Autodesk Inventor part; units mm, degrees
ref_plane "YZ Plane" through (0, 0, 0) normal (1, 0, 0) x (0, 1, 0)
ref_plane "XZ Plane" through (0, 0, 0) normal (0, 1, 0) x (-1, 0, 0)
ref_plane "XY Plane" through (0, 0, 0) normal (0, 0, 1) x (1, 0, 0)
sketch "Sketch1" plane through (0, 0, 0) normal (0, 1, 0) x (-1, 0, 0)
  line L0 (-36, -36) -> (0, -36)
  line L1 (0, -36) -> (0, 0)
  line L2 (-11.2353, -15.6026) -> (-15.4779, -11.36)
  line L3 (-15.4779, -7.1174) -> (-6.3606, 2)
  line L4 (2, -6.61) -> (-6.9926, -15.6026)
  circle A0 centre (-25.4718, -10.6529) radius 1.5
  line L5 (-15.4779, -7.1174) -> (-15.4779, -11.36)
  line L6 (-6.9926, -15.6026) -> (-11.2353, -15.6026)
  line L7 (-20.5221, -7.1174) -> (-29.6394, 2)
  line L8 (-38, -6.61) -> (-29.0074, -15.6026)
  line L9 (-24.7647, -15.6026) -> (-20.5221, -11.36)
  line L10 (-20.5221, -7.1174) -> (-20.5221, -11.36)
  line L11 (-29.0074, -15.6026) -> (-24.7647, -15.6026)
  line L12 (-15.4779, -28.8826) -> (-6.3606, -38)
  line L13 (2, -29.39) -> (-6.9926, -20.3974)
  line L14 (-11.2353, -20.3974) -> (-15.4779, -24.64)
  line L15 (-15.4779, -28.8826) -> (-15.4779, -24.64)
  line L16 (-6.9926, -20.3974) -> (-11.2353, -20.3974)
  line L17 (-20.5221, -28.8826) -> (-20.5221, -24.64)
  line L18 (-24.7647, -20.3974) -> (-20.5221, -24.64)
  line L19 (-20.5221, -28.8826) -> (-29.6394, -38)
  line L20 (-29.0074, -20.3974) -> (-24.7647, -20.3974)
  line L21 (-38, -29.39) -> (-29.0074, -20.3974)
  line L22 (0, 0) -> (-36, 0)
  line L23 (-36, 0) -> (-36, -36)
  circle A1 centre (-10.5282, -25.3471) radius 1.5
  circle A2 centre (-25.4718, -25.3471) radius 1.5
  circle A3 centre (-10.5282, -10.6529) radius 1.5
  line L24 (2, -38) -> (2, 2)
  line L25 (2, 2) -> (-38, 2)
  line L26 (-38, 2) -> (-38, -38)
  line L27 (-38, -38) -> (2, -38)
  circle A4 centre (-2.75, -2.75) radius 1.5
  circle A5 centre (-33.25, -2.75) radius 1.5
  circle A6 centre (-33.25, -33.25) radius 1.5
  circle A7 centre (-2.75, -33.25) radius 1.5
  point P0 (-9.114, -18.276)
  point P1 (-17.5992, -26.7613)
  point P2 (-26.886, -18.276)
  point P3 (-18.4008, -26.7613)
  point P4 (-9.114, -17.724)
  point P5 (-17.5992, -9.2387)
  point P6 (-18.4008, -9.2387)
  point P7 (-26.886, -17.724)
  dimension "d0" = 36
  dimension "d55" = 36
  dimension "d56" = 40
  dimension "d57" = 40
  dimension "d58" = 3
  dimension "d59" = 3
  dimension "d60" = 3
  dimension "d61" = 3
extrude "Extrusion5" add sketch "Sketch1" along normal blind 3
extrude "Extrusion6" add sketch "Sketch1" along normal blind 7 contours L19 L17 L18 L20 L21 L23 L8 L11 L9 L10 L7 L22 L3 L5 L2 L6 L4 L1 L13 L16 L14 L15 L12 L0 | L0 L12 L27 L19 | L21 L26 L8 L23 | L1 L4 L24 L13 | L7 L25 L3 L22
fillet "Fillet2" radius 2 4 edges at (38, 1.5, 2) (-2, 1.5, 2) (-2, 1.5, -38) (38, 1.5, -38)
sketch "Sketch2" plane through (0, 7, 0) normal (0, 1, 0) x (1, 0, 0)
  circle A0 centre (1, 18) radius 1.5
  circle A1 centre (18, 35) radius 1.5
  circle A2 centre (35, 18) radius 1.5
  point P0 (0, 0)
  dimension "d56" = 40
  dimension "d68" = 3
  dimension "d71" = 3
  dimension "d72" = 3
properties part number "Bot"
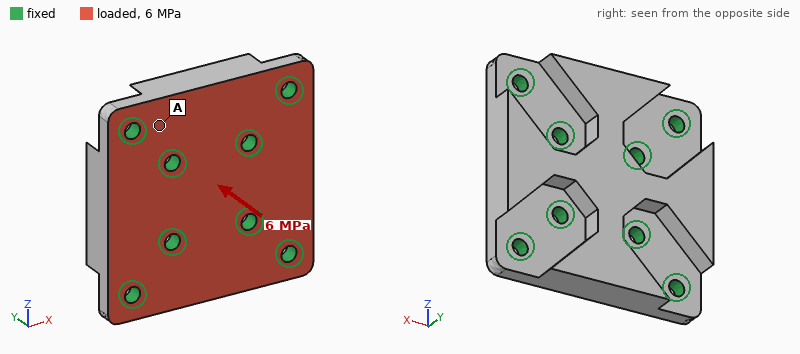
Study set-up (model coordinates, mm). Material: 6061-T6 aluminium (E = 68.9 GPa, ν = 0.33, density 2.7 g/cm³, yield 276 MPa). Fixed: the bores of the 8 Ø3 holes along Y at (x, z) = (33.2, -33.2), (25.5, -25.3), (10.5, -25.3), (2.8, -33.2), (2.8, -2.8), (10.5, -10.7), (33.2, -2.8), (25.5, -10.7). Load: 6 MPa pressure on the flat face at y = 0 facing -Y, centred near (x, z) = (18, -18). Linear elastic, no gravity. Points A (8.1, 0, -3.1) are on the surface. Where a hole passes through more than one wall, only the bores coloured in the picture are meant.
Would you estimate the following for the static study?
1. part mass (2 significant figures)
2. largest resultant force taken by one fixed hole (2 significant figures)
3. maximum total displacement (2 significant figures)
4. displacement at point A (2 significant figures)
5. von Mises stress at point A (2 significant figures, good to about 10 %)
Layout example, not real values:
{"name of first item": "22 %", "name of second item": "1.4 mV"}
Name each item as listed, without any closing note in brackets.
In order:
{"part mass": "20 g", "largest resultant force taken by one fixed hole": "1.3 kN", "maximum total displacement": "19 µm", "displacement at point A": "7.2 µm", "von Mises stress at point A": "32 MPa"}
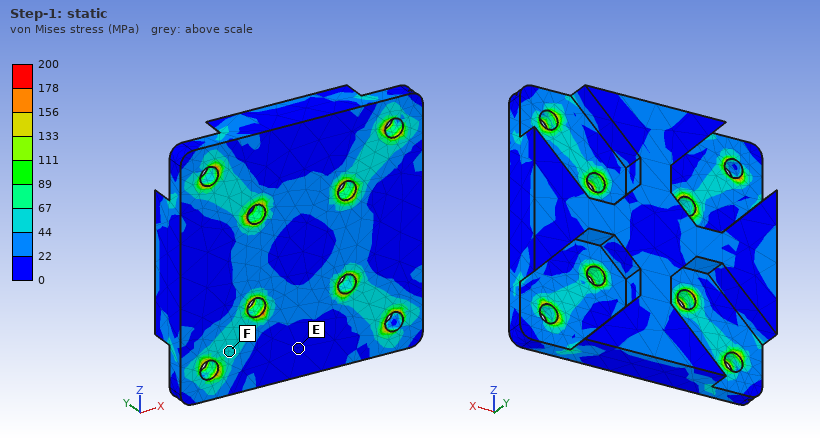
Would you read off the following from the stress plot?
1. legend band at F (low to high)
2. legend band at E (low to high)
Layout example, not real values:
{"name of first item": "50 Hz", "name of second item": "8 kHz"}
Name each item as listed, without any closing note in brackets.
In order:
{"legend band at F": "44 to 67 MPa", "legend band at E": "0 to 22 MPa"}
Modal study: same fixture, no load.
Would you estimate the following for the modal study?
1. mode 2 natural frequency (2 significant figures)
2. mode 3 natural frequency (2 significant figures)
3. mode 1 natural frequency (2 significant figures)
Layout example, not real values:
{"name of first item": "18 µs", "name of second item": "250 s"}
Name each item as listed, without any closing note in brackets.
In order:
{"mode 2 natural frequency": "25 kHz", "mode 3 natural frequency": "25 kHz", "mode 1 natural frequency": "24 kHz"}
